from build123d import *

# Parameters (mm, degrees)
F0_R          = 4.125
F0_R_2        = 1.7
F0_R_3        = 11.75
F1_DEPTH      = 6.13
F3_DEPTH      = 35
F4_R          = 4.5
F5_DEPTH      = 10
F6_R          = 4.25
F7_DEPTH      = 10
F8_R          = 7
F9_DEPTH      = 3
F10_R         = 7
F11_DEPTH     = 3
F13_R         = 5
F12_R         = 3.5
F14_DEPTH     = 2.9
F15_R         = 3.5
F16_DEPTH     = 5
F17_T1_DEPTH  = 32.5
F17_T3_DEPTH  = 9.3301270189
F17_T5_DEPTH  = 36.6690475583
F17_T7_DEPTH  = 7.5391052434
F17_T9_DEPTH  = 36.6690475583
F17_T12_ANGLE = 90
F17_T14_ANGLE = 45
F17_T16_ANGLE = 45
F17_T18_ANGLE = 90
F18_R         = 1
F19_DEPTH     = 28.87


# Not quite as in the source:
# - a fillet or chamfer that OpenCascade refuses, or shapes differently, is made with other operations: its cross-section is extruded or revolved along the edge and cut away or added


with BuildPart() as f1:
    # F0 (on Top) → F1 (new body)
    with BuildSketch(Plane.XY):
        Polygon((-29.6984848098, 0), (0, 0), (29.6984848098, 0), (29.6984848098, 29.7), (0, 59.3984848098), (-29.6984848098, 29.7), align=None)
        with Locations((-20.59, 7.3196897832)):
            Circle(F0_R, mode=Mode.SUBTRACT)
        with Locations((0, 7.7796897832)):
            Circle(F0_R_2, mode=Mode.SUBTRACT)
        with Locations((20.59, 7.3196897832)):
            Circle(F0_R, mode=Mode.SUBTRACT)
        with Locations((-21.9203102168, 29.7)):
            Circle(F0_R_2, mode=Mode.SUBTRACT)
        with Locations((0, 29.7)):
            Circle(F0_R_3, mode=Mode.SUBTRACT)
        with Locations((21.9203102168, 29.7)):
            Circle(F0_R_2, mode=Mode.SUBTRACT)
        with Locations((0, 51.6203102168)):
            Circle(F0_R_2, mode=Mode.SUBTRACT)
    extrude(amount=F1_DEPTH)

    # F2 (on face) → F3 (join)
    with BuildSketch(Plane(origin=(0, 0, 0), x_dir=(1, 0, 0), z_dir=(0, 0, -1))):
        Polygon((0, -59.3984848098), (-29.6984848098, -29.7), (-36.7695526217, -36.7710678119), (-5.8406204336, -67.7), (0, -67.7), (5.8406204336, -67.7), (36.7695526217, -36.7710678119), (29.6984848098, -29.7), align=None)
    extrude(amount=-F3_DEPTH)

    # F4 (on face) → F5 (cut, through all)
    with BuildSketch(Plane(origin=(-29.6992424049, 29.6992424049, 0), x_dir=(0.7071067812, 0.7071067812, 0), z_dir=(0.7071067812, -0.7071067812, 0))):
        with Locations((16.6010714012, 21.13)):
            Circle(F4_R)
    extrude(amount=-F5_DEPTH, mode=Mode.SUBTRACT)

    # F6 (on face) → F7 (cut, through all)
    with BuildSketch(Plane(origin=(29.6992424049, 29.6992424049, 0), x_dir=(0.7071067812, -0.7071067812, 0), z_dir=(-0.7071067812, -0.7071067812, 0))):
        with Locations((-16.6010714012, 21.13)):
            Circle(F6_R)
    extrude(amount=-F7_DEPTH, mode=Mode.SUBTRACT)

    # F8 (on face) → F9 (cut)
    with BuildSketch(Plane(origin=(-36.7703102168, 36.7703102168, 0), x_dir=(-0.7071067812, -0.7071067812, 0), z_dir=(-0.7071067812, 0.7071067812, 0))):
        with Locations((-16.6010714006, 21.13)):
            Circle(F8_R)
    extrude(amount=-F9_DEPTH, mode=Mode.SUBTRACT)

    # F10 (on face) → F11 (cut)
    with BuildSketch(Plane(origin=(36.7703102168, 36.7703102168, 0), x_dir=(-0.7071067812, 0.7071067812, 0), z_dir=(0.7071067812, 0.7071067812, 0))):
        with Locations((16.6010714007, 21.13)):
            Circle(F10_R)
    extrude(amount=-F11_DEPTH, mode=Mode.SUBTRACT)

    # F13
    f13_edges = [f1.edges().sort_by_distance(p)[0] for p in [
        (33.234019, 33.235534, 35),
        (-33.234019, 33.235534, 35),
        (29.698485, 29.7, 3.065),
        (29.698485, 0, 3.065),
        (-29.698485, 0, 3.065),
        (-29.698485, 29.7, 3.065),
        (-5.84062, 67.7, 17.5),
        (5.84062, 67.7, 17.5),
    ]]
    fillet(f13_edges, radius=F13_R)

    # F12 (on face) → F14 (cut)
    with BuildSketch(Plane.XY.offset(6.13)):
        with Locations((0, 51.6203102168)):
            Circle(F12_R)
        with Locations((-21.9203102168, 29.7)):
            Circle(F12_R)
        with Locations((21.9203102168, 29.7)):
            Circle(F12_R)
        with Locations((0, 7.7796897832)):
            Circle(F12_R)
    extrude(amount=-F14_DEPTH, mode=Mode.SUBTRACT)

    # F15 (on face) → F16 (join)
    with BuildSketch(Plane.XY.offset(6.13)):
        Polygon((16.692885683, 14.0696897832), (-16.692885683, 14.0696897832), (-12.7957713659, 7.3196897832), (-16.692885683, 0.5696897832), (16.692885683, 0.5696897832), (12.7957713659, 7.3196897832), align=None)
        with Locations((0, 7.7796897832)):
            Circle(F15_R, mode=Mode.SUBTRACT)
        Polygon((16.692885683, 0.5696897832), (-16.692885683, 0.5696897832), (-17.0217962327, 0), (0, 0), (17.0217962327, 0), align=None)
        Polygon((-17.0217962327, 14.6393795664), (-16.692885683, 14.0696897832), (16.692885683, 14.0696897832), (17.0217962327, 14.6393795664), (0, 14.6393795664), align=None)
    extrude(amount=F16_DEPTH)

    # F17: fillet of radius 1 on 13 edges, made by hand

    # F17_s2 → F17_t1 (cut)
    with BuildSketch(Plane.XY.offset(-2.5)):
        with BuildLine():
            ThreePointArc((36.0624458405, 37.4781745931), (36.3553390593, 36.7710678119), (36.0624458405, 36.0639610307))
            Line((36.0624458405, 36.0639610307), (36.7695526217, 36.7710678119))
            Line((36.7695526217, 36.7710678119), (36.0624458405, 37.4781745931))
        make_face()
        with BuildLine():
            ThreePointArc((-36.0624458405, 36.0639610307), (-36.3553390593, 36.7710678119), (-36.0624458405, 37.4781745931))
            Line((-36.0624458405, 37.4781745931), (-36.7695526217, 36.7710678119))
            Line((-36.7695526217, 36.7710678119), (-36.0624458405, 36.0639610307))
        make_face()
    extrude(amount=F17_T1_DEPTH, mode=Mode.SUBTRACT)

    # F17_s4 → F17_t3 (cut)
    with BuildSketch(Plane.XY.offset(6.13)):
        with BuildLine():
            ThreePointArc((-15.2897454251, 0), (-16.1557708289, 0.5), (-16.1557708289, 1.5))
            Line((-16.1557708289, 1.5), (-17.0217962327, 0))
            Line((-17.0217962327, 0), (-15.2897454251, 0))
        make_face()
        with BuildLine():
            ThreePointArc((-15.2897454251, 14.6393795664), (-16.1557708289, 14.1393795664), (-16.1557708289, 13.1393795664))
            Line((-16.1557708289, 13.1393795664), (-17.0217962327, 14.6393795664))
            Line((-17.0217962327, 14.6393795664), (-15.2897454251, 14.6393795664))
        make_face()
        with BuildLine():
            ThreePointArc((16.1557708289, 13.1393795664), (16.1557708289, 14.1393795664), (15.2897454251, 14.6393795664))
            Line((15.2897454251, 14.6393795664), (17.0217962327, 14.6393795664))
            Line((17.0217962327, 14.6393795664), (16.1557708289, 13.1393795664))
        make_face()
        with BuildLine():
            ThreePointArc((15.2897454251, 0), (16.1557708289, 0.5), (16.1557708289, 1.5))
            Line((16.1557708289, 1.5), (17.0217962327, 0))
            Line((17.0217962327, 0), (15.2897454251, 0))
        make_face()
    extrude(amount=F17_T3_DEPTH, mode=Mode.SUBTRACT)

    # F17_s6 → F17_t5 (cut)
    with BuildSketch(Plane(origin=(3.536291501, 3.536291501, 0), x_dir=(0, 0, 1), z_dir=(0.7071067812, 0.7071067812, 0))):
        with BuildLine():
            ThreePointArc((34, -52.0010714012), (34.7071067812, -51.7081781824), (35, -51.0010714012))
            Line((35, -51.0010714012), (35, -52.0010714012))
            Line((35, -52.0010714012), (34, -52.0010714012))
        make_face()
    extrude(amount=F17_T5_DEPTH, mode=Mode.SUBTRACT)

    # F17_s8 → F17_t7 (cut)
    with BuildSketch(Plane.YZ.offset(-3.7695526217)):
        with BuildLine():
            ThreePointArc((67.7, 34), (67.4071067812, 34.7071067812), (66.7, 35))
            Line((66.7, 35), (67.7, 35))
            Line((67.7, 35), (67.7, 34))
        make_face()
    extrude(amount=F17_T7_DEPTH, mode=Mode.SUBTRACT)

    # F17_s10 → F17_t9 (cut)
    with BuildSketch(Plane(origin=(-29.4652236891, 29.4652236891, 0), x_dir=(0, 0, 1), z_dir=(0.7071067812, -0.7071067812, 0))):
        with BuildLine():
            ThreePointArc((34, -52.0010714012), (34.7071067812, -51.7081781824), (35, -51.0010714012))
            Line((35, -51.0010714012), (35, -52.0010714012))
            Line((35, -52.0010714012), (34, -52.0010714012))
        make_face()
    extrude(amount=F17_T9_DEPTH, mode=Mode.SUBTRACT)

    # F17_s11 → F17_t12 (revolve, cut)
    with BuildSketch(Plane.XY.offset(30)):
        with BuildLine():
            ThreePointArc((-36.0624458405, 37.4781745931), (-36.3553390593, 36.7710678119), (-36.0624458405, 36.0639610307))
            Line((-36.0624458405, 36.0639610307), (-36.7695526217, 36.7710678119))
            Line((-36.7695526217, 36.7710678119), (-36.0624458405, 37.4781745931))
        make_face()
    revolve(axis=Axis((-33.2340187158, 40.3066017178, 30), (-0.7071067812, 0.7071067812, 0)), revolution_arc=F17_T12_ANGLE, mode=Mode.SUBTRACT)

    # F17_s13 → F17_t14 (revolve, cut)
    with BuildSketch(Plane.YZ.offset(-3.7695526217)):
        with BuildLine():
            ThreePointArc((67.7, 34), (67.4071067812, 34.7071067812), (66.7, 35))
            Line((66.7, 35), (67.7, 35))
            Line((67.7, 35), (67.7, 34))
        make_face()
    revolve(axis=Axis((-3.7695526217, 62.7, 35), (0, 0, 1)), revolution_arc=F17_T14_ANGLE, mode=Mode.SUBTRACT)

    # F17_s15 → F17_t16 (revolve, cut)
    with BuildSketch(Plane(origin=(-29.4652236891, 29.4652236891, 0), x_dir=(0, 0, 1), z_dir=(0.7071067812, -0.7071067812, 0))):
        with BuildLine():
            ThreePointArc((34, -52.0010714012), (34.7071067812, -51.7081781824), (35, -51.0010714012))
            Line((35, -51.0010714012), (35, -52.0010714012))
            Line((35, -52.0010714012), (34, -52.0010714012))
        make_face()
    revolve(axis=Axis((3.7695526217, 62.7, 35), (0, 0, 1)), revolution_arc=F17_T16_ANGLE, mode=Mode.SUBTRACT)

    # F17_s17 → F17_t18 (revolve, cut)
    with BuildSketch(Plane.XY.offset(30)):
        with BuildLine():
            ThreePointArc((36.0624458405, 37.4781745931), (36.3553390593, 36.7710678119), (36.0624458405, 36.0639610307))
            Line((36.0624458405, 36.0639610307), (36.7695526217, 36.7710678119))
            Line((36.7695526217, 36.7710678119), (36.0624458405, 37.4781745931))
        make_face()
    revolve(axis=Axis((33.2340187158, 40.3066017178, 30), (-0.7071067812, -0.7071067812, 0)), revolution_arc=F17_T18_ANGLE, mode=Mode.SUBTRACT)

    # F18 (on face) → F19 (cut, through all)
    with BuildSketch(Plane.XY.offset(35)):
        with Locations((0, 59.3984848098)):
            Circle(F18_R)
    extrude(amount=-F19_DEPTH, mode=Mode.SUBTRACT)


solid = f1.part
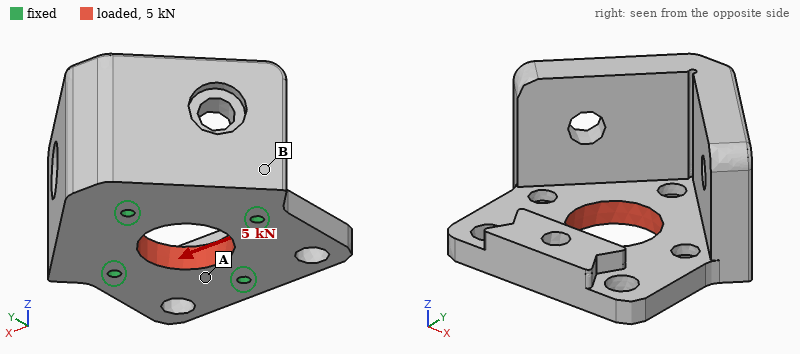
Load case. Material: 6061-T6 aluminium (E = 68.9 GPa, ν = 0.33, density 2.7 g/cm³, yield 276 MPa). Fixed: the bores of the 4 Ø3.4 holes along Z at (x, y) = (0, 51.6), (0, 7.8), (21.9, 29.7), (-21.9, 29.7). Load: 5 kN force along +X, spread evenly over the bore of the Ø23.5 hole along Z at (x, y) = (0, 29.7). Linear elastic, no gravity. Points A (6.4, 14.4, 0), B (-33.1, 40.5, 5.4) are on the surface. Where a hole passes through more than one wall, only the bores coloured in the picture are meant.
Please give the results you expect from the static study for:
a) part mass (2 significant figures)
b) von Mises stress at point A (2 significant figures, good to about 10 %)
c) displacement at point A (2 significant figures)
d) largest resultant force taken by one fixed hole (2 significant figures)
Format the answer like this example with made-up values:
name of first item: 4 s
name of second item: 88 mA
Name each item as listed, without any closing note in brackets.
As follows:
part mass: 120 g
von Mises stress at point A: 12 MPa
displacement at point A: 3.3 µm
largest resultant force taken by one fixed hole: 1.3 kN
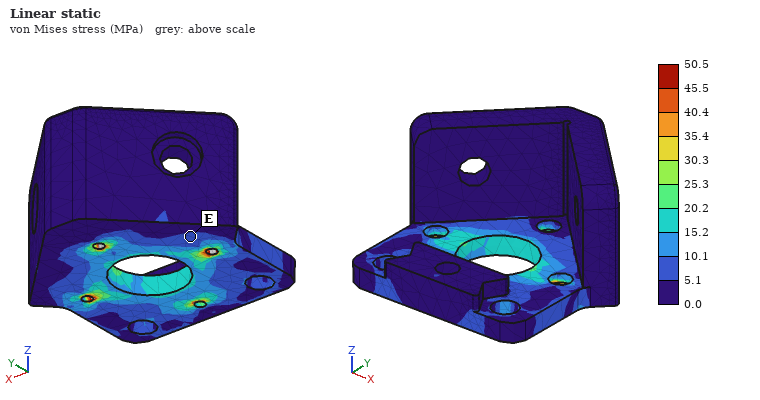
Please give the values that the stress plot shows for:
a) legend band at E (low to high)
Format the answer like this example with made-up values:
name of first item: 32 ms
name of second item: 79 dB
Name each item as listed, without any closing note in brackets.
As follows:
legend band at E: 5.1 to 10.1 MPa
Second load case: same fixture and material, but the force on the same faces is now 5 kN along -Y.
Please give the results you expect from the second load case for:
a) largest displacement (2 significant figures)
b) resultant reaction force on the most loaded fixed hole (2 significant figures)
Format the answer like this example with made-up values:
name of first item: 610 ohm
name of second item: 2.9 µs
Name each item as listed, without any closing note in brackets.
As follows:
largest displacement: 5.0 µm
resultant reaction force on the most loaded fixed hole: 1.4 kN
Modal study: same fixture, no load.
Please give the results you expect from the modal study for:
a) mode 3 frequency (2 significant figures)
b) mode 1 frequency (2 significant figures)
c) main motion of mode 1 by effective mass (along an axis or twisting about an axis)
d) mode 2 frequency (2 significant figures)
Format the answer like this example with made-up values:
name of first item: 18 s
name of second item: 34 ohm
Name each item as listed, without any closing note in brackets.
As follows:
mode 3 frequency: 7600 Hz
mode 1 frequency: 3900 Hz
main motion of mode 1 by effective mass: along X
mode 2 frequency: 4800 Hz
